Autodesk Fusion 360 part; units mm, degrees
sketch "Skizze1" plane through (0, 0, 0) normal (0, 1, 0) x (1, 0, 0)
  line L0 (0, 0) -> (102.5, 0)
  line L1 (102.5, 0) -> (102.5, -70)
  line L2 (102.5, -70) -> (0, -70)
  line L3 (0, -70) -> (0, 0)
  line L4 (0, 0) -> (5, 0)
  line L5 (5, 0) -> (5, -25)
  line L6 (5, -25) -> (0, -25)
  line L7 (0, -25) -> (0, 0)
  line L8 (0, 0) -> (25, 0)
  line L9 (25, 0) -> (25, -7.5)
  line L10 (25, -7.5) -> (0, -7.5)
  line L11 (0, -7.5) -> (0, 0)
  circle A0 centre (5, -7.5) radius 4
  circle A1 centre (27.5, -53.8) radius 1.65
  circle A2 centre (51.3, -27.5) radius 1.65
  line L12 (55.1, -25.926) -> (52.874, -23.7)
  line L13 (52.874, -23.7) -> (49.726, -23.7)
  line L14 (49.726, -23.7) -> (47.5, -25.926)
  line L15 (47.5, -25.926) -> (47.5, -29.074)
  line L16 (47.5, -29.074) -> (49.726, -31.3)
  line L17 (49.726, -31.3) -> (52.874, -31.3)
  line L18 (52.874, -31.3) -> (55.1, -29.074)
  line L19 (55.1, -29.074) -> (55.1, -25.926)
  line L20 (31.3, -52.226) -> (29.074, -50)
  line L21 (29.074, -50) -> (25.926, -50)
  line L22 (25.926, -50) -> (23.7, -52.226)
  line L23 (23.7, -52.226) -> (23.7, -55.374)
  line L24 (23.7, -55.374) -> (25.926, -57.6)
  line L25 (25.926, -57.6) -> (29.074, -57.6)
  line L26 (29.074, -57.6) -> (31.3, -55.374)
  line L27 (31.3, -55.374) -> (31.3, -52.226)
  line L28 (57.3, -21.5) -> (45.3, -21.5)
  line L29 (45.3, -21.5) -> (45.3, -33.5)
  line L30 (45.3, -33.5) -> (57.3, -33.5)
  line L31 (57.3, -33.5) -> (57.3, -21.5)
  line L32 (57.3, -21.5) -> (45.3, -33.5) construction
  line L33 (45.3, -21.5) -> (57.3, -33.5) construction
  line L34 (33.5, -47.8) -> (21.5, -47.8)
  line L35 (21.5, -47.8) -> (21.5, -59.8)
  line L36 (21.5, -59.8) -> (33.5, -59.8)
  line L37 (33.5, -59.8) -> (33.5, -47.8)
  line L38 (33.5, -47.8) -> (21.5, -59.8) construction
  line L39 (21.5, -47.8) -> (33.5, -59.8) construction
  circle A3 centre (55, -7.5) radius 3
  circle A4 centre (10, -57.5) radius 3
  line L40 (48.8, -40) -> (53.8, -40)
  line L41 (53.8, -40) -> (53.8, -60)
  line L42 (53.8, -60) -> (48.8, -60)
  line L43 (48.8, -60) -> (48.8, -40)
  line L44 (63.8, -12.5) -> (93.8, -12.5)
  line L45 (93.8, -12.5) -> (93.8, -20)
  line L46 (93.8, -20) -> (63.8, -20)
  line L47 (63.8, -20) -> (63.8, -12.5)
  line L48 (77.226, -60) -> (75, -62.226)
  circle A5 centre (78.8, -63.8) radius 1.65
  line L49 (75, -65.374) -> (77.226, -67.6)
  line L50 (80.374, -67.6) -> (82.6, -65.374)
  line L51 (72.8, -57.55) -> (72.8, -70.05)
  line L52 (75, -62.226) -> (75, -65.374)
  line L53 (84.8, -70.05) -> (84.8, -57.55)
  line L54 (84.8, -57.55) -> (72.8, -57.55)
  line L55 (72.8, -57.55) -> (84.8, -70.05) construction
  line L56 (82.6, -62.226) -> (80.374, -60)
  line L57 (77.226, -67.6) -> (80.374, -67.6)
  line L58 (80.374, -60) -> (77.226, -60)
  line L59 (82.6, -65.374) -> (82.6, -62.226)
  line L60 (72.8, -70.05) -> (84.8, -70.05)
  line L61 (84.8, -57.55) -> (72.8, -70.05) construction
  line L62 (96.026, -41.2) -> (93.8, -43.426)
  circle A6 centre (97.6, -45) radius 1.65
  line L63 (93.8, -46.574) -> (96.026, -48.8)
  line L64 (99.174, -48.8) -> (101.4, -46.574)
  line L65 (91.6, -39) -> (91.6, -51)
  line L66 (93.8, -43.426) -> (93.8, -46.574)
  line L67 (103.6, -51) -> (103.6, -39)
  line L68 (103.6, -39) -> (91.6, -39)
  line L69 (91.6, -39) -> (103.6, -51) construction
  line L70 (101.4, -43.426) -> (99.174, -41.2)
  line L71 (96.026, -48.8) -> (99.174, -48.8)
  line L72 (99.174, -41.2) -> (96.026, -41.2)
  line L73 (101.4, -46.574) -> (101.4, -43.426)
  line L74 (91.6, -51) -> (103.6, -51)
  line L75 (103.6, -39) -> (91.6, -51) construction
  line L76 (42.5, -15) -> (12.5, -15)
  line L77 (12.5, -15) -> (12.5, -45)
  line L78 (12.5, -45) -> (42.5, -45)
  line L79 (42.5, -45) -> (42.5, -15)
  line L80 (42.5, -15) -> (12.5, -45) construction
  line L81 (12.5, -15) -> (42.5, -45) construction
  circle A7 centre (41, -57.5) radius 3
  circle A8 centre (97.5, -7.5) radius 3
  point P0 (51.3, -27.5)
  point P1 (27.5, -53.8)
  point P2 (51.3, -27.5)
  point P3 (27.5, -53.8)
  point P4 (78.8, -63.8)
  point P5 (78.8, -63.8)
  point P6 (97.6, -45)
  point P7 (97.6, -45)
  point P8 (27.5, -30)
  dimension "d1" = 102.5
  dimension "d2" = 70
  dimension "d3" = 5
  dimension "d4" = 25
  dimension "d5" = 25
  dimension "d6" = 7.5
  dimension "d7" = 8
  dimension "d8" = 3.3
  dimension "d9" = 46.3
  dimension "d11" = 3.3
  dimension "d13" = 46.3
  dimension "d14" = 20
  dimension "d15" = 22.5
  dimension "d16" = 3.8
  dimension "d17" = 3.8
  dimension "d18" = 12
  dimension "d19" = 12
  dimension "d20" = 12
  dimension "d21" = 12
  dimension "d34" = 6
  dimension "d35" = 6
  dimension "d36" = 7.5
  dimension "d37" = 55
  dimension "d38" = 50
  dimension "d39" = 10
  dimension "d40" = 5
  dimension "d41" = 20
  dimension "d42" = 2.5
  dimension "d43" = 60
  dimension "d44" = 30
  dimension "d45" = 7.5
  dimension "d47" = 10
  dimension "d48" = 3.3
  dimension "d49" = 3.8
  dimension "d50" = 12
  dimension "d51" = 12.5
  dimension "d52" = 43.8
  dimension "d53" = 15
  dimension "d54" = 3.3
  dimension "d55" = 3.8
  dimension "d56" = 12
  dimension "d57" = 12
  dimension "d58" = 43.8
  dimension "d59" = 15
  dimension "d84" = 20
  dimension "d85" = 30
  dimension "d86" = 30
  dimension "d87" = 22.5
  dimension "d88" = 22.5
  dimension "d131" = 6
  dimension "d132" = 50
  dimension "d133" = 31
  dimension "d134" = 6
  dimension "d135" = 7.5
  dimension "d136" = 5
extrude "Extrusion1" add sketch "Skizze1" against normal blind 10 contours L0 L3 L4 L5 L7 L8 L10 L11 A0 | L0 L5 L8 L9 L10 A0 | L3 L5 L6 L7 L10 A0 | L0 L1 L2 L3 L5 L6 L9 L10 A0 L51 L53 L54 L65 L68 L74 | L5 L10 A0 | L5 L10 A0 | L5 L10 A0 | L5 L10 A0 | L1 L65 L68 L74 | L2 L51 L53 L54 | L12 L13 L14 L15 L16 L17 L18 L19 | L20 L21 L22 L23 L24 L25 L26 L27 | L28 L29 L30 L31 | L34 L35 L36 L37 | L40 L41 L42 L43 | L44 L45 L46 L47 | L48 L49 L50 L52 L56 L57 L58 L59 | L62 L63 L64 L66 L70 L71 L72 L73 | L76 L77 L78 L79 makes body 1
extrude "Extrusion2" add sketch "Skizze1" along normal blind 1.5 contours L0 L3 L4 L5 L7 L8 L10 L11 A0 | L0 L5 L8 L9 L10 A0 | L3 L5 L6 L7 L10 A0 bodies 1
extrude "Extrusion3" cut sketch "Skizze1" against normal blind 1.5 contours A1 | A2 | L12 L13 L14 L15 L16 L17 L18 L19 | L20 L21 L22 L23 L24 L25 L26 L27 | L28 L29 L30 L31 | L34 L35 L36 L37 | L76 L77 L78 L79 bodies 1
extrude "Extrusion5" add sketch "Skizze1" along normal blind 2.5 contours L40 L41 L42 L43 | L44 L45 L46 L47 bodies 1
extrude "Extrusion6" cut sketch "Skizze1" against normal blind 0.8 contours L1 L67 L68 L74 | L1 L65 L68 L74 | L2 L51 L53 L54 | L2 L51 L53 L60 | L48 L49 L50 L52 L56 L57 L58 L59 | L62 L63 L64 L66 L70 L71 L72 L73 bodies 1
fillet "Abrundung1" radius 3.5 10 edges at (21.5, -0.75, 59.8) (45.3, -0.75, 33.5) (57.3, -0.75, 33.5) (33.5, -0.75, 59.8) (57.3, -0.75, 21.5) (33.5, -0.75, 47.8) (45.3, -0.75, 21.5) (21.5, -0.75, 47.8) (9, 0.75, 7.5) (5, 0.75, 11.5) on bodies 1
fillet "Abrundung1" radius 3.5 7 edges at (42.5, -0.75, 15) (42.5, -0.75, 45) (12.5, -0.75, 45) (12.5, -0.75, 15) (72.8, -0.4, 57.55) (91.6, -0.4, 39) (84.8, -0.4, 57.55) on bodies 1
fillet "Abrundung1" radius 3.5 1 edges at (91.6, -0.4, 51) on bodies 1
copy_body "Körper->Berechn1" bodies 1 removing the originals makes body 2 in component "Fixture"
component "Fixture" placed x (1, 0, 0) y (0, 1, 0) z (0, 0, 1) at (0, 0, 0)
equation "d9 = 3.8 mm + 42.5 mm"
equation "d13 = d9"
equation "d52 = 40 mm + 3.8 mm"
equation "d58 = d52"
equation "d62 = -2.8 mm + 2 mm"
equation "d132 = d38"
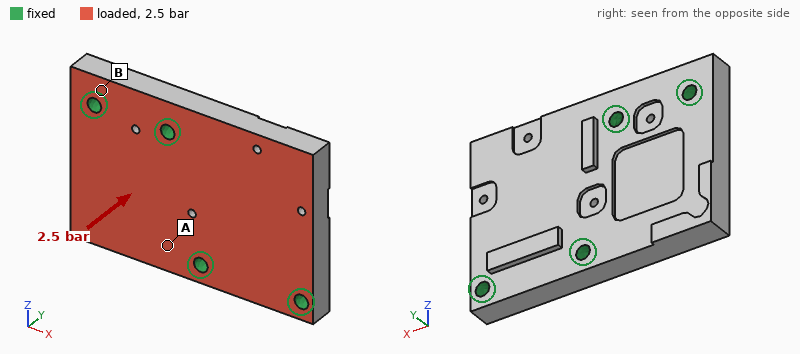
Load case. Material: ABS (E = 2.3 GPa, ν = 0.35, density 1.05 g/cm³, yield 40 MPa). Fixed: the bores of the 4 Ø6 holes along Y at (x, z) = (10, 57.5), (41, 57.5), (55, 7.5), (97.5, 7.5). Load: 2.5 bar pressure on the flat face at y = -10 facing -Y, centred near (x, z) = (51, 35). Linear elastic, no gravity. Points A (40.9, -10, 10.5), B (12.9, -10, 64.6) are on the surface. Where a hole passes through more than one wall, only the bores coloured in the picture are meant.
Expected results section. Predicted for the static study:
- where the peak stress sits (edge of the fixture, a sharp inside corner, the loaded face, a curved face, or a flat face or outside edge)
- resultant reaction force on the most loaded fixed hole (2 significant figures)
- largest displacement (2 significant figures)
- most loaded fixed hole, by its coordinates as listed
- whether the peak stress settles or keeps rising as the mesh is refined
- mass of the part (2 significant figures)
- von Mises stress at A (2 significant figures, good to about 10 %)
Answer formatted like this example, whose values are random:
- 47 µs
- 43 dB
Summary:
- edge of the fixture
- 600 N
- 0.90 mm
- (41, 57.5)
- keeps rising
- 73 g
- 5.6 MPa
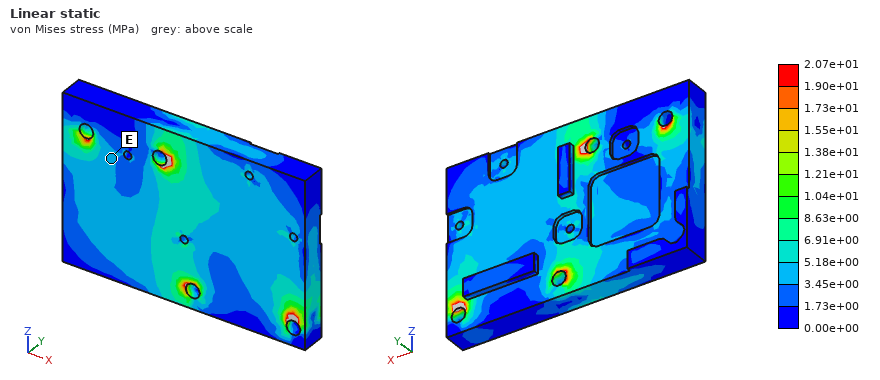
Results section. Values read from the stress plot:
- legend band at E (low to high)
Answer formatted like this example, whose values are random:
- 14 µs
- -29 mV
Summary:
- 3.45e+00 to 5.18e+00 MPa
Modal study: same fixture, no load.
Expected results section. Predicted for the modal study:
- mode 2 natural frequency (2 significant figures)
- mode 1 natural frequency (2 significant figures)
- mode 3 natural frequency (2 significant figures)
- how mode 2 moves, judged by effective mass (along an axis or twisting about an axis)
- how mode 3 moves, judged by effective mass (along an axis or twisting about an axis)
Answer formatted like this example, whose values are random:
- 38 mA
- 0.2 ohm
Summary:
- 1300 Hz
- 1100 Hz
- 3500 Hz
- along Y
- along Y
